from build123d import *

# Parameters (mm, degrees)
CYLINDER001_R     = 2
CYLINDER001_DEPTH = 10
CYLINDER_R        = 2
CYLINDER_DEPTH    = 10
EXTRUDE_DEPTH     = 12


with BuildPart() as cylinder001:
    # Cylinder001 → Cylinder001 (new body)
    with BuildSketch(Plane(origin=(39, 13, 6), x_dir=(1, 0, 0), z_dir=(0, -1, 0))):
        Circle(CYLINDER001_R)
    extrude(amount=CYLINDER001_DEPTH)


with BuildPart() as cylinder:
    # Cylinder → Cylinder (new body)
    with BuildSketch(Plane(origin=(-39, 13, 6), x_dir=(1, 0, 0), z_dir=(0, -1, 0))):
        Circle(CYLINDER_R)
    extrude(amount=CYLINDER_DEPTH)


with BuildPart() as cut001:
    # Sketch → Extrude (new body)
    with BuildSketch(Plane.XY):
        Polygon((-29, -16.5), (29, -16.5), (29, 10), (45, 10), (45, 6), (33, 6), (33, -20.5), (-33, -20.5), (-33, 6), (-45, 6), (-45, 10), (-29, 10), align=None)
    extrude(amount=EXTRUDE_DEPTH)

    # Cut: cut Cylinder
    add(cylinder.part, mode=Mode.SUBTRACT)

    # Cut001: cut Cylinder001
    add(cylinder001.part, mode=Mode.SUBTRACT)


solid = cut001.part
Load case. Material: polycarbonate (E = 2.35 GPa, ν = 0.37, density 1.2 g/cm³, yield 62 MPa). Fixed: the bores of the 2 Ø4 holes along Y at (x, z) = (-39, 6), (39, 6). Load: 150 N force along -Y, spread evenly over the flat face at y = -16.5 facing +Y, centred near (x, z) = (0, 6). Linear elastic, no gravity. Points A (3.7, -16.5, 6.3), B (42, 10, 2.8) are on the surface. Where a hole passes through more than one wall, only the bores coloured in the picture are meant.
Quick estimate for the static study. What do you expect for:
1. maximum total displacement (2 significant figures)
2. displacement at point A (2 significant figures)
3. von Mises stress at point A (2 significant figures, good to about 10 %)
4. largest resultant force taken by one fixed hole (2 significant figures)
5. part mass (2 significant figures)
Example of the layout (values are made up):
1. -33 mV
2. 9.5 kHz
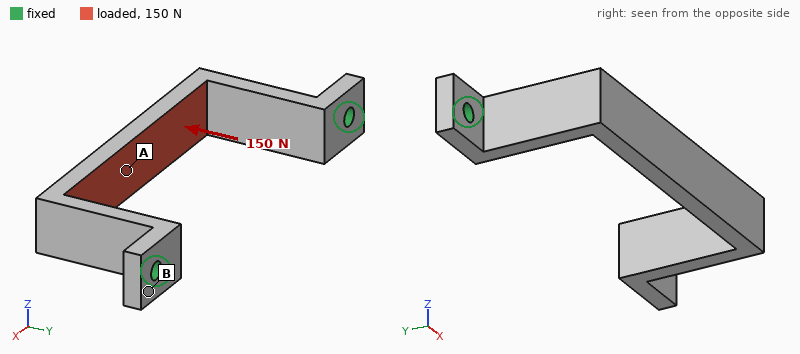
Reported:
1. 1.1 mm
2. 1.0 mm
3. 15 MPa
4. 85 N
5. 8.1 g
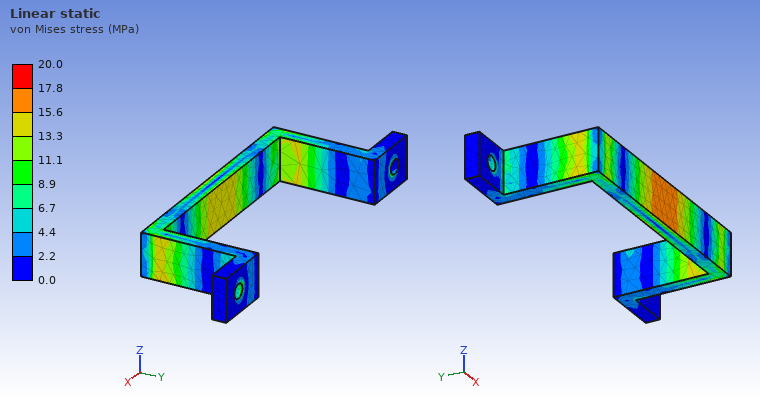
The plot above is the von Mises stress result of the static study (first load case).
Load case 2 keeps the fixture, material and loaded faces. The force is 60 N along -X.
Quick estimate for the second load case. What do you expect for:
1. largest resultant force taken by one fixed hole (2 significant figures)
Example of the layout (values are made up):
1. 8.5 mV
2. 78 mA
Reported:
1. 32 N
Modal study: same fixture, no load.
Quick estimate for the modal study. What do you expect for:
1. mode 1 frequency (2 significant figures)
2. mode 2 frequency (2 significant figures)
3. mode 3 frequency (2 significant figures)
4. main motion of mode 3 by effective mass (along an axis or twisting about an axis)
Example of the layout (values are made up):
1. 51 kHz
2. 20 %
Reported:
1. 650 Hz
2. 650 Hz
3. 1100 Hz
4. twisting about Y
